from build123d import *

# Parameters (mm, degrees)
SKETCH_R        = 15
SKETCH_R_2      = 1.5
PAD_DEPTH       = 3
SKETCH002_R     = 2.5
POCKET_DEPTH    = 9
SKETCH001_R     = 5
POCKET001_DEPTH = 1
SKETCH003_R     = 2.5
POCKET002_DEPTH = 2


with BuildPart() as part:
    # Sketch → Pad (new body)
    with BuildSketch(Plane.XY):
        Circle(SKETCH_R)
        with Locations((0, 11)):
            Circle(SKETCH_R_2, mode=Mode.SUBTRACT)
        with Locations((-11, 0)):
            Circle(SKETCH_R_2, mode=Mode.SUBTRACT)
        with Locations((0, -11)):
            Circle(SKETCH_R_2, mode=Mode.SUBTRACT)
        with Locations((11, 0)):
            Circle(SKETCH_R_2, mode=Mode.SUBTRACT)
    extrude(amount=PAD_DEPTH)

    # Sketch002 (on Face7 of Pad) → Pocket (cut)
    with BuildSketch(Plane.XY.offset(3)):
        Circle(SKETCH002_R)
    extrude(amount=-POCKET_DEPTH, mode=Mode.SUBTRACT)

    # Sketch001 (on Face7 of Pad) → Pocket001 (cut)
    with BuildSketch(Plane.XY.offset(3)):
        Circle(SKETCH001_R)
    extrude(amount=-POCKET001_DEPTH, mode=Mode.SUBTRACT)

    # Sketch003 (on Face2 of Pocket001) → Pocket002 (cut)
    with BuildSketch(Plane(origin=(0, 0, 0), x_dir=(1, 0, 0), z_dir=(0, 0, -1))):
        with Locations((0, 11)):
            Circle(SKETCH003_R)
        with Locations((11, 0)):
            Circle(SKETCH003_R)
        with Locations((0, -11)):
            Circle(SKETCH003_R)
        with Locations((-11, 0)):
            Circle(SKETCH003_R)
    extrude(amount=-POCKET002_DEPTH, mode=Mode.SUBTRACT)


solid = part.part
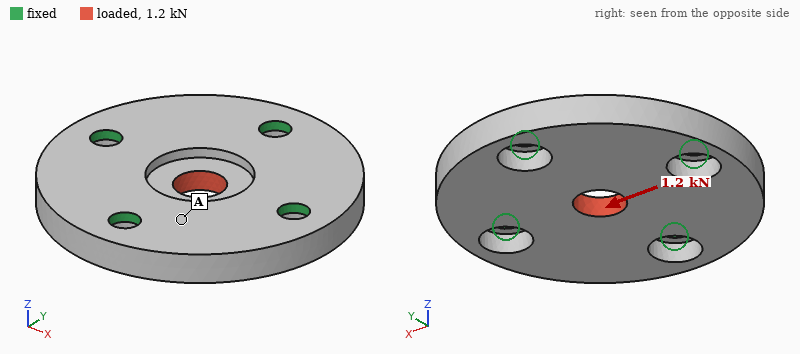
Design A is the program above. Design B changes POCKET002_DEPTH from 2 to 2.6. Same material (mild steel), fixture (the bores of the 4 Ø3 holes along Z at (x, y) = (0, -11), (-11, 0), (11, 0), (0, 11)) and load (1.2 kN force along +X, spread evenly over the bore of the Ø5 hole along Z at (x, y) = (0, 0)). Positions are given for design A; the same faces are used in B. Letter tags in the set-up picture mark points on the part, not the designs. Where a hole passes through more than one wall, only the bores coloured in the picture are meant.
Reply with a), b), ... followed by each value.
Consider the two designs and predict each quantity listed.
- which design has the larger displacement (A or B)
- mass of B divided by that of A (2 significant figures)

a) B
b) 0.98
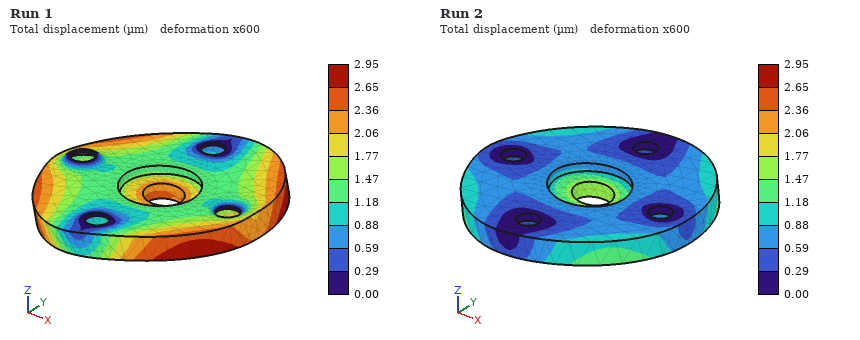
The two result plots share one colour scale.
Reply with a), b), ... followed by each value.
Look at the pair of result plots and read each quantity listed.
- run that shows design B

a) Run 1
